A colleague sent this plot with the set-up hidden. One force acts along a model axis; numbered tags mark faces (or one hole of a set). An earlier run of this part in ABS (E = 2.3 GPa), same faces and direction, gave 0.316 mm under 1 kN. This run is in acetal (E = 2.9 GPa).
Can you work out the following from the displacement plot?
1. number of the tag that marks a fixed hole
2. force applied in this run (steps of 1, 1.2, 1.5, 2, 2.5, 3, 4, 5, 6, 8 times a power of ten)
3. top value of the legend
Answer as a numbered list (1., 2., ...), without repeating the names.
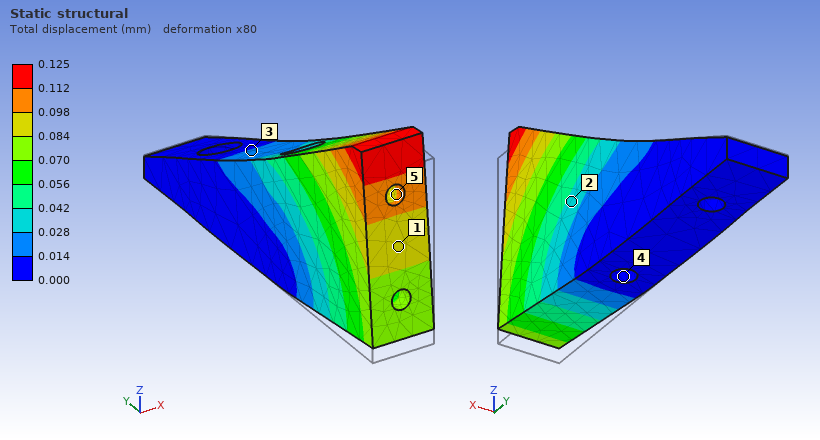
1. 4
2. 500 N
3. 0.125 mm
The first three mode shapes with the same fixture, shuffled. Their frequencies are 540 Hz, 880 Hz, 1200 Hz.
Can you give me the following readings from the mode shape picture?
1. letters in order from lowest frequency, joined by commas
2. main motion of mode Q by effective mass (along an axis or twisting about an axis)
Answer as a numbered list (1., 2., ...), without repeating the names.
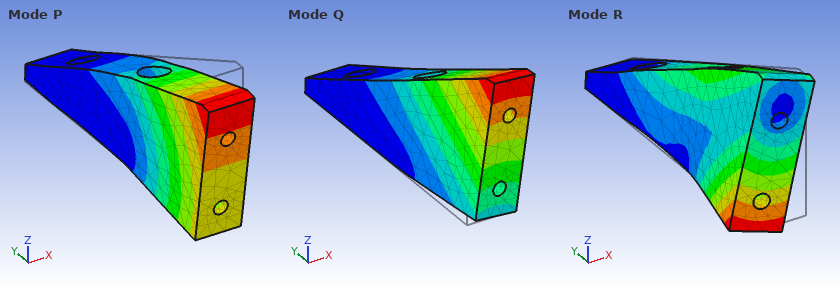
1. Q, P, R
2. along X
